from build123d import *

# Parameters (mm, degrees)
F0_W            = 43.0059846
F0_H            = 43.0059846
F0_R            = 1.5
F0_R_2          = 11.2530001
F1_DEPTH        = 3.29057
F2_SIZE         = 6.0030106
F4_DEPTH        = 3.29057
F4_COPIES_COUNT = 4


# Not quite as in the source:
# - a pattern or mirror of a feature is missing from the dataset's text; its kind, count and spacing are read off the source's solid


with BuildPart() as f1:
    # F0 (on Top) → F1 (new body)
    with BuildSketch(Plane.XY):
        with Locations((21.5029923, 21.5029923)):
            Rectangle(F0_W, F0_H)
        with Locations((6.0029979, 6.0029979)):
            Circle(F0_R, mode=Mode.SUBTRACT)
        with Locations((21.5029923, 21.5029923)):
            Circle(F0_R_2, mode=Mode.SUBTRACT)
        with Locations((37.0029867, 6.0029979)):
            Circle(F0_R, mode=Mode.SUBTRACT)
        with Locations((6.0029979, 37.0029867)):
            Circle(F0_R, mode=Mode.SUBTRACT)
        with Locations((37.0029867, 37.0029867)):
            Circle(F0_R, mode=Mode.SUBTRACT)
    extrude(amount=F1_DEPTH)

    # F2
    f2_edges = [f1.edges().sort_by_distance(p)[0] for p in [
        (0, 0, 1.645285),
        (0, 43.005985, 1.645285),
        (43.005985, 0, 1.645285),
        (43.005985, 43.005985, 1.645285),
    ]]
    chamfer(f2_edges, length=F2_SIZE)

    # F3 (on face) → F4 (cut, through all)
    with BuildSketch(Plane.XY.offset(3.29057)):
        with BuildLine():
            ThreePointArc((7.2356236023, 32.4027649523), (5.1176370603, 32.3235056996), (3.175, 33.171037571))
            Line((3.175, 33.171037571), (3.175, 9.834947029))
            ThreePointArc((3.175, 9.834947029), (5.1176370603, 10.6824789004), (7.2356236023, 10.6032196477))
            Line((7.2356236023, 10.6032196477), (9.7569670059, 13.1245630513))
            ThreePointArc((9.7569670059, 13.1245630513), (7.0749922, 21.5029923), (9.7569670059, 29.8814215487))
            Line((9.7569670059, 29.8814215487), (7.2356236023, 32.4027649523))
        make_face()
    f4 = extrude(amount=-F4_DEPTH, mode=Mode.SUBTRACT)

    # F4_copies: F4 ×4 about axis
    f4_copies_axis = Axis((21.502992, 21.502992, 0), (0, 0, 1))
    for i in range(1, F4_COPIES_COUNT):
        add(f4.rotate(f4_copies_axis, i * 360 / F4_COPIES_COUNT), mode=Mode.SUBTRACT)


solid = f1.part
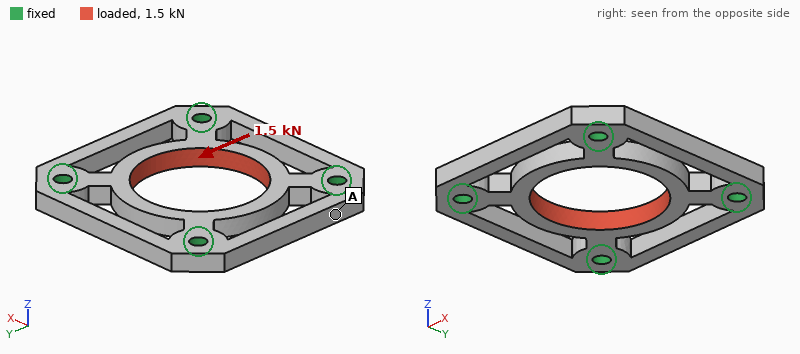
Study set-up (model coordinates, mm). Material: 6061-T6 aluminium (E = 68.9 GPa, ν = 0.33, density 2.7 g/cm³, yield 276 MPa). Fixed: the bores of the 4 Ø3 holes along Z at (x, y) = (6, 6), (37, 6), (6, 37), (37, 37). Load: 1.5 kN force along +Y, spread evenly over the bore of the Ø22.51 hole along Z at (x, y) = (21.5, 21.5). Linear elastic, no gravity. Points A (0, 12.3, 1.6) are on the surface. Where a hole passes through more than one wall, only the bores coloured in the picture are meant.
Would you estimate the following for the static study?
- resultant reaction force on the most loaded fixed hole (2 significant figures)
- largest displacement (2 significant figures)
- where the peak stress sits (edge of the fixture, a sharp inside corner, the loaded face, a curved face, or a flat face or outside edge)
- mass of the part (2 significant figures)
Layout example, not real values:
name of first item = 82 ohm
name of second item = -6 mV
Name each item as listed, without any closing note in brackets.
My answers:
resultant reaction force on the most loaded fixed hole = 380 N
largest displacement = 31 µm
where the peak stress sits = edge of the fixture
mass of the part = 8.2 g
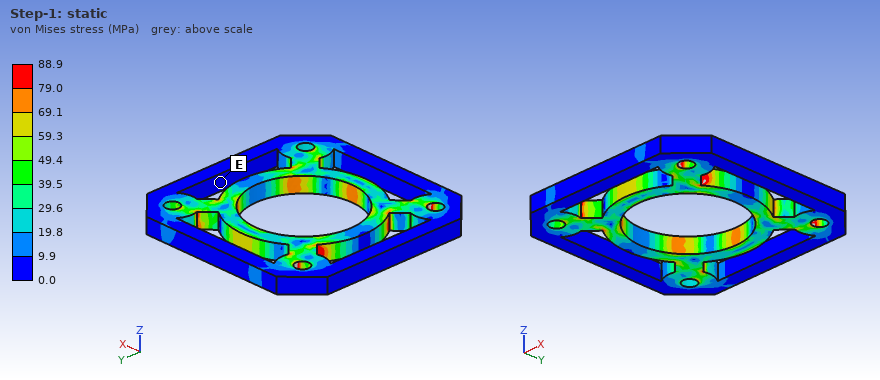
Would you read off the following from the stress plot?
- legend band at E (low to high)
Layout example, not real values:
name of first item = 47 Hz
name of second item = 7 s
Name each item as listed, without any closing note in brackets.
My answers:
legend band at E = 0.0 to 9.9 MPa
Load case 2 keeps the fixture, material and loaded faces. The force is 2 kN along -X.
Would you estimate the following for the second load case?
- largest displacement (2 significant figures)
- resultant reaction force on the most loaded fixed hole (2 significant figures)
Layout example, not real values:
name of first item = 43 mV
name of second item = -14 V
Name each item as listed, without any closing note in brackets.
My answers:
largest displacement = 41 µm
resultant reaction force on the most loaded fixed hole = 500 N
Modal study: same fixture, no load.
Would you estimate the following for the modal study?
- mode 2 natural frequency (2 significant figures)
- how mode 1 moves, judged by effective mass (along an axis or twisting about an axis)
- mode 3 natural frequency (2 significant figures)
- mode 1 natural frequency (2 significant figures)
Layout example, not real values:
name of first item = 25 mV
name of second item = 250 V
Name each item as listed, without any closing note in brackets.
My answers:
mode 2 natural frequency = 17 kHz
how mode 1 moves, judged by effective mass = along Z
mode 3 natural frequency = 18 kHz
mode 1 natural frequency = 16 kHz
